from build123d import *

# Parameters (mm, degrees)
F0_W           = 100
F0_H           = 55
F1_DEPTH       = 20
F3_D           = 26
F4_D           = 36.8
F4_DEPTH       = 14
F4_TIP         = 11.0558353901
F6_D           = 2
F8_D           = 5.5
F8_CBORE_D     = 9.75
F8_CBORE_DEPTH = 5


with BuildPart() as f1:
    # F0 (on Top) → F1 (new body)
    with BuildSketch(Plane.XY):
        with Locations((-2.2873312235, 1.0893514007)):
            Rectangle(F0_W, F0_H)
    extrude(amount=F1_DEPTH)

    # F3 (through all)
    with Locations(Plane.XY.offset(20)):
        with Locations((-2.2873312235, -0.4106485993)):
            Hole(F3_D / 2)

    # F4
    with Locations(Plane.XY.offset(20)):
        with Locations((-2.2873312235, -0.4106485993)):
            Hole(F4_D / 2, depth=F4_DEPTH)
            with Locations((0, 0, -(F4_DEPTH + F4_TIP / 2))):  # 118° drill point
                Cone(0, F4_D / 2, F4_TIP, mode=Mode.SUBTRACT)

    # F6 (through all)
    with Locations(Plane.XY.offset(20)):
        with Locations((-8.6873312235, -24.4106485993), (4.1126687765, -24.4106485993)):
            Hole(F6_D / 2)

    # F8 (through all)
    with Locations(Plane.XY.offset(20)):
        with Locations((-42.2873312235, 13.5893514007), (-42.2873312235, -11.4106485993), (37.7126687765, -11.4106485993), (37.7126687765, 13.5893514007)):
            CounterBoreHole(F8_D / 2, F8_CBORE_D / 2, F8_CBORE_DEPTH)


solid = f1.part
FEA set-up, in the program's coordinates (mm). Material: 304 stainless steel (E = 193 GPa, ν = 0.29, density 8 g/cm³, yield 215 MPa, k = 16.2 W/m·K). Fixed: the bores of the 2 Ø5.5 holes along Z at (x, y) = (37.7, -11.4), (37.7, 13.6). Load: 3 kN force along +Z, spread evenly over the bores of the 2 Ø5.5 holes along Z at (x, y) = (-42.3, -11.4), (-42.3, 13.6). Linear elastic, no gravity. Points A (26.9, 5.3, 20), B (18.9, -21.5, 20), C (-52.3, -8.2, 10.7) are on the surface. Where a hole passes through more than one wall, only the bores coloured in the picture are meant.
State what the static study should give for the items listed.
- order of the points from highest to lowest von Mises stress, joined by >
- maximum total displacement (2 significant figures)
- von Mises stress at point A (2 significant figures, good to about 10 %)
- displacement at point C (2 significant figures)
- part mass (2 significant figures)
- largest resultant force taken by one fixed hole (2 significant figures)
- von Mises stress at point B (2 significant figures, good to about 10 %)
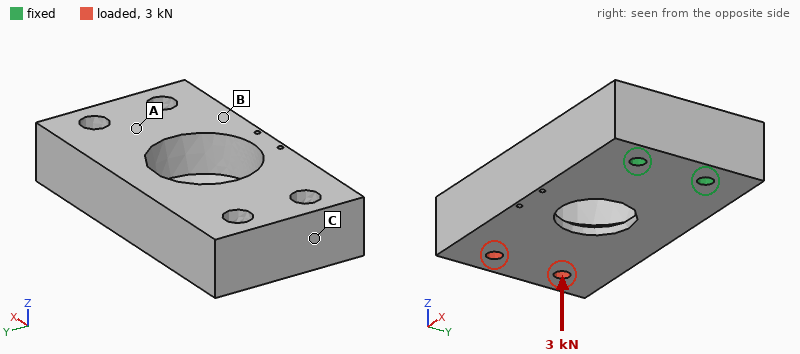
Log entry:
B > A > C
0.18 mm
39 MPa
0.18 mm
700 g
1.6 kN
76 MPa
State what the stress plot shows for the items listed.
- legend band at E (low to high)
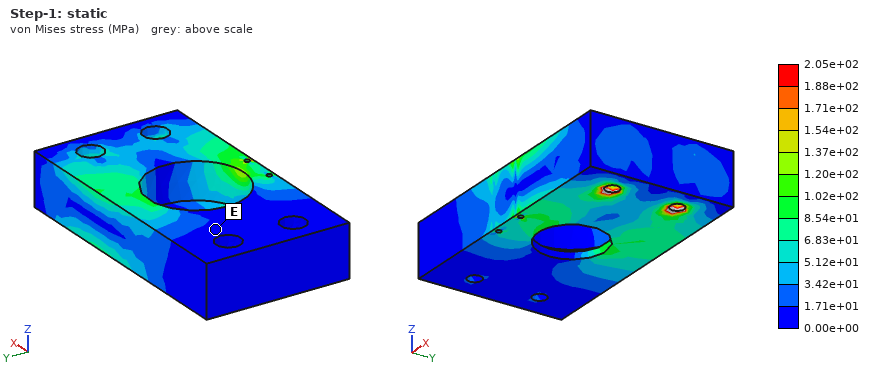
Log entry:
0.00e+00 to 1.71e+01 MPa
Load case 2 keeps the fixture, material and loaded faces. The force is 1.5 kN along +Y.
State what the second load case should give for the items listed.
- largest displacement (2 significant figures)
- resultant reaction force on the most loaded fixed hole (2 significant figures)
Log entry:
19 µm
4.2 kN
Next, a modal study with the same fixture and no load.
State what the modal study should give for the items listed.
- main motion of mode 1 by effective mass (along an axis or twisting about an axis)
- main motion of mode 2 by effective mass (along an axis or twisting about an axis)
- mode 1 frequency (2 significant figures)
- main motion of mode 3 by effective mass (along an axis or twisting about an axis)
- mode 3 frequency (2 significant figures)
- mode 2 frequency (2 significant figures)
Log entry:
along Z
along Y
1400 Hz
twisting about X
4200 Hz
2800 Hz
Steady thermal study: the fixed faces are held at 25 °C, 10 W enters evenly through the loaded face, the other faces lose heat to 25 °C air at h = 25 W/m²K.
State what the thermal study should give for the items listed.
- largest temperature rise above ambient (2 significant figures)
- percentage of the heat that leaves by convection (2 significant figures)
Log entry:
37 K
70 %
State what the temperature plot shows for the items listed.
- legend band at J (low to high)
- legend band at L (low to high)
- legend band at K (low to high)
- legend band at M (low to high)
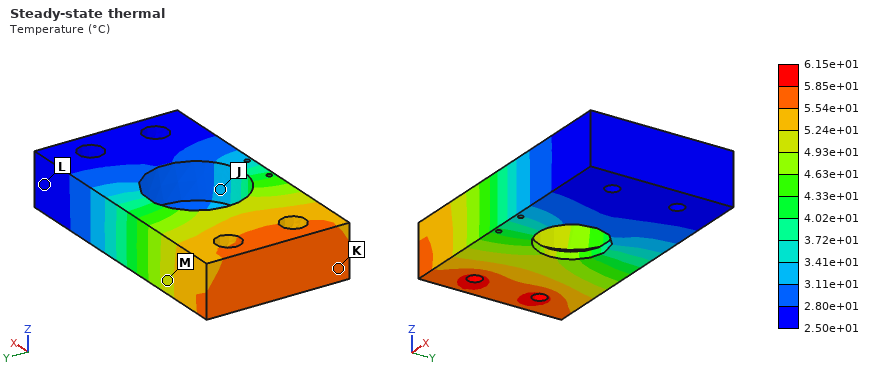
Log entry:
3.11e+01 to 3.41e+01 °C
2.50e+01 to 2.80e+01 °C
5.54e+01 to 5.85e+01 °C
4.93e+01 to 5.24e+01 °C
